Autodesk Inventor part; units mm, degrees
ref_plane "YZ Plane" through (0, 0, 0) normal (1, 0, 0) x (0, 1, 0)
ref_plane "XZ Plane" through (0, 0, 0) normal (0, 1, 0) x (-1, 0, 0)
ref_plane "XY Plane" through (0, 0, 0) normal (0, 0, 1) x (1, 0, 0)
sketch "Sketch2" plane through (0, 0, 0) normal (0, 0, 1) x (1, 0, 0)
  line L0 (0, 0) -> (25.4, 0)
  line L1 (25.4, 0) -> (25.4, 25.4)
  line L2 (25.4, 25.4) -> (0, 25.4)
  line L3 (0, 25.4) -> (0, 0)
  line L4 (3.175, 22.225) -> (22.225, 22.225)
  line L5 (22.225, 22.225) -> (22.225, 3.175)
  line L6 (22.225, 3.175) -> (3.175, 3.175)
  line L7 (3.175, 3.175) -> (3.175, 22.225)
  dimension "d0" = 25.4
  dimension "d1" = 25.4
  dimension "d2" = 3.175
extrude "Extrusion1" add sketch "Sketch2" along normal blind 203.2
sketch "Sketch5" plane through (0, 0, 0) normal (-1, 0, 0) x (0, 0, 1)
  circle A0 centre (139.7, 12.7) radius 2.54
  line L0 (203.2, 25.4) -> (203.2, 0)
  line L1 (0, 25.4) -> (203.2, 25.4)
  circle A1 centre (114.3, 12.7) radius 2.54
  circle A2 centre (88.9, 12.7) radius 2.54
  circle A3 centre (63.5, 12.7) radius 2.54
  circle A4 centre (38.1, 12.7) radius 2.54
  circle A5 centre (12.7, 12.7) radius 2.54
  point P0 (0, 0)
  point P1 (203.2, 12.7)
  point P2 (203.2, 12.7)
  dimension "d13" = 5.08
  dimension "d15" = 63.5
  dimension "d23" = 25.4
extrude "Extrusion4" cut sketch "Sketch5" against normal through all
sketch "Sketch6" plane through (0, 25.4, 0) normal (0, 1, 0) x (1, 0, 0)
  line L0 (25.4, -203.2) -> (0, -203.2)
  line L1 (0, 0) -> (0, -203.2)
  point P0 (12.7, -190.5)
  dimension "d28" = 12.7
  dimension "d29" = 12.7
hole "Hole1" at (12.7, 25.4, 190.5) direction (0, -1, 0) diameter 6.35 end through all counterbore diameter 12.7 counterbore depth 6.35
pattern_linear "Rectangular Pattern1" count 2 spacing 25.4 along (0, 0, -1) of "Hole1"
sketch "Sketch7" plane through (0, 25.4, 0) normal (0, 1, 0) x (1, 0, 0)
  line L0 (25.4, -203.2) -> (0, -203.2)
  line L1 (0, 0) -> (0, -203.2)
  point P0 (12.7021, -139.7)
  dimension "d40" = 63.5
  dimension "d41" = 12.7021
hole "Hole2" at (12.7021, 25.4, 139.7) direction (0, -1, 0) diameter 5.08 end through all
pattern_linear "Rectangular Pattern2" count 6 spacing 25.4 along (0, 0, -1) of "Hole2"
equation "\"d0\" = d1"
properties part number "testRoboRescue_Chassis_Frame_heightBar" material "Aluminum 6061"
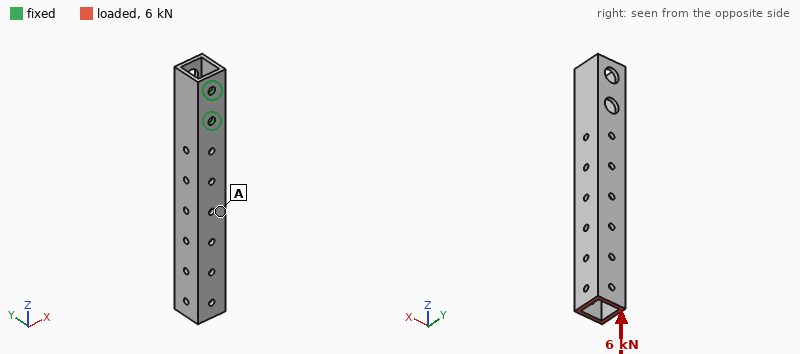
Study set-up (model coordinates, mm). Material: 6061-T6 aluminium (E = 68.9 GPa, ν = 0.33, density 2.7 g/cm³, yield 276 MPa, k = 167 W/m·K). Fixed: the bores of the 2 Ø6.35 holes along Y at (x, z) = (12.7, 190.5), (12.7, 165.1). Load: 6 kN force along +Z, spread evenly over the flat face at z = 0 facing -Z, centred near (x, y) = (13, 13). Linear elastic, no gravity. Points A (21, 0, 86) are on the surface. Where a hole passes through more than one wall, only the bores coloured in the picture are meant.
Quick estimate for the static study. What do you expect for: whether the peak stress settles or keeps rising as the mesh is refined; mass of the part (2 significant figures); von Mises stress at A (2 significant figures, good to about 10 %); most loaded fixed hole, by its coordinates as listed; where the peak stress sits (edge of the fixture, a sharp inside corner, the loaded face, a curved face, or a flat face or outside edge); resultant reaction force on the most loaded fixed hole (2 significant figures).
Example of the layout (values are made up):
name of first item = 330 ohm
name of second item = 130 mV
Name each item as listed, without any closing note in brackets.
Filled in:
whether the peak stress settles or keeps rising as the mesh is refined = keeps rising
mass of the part = 150 g
von Mises stress at A = 24 MPa
most loaded fixed hole, by its coordinates as listed = (12.7, 165.1)
where the peak stress sits = edge of the fixture
resultant reaction force on the most loaded fixed hole = 4.3 kN
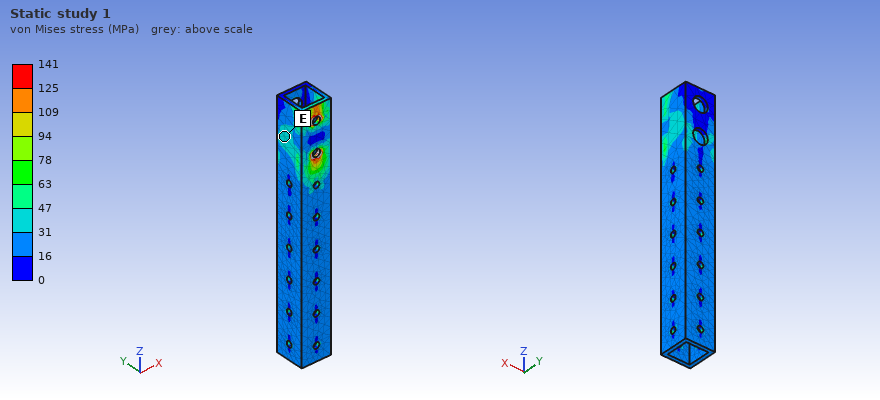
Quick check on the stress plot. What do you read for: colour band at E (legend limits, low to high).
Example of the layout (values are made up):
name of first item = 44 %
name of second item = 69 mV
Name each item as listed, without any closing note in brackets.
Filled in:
colour band at E = 31 to 47 MPa
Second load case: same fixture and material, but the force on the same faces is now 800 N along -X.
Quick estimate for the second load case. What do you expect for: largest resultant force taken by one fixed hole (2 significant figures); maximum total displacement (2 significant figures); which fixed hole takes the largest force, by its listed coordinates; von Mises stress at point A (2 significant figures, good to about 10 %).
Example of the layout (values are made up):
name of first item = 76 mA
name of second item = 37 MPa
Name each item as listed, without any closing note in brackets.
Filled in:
largest resultant force taken by one fixed hole = 4.5 kN
maximum total displacement = 1.5 mm
which fixed hole takes the largest force, by its listed coordinates = (12.7, 165.1)
von Mises stress at point A = 22 MPa
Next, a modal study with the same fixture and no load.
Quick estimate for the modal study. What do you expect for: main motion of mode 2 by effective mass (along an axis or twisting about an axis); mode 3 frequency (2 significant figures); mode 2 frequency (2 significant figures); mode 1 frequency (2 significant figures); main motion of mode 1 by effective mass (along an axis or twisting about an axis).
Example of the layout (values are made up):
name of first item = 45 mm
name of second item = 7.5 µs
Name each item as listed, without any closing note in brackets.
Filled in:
main motion of mode 2 by effective mass = along X
mode 3 frequency = 1700 Hz
mode 2 frequency = 630 Hz
mode 1 frequency = 500 Hz
main motion of mode 1 by effective mass = along Y
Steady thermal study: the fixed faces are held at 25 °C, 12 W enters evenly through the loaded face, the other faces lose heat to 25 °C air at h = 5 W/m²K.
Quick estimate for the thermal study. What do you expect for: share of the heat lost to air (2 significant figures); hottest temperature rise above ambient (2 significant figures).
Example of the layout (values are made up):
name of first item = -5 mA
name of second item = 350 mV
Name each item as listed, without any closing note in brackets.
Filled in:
share of the heat lost to air = 26 %
hottest temperature rise above ambient = 41 K
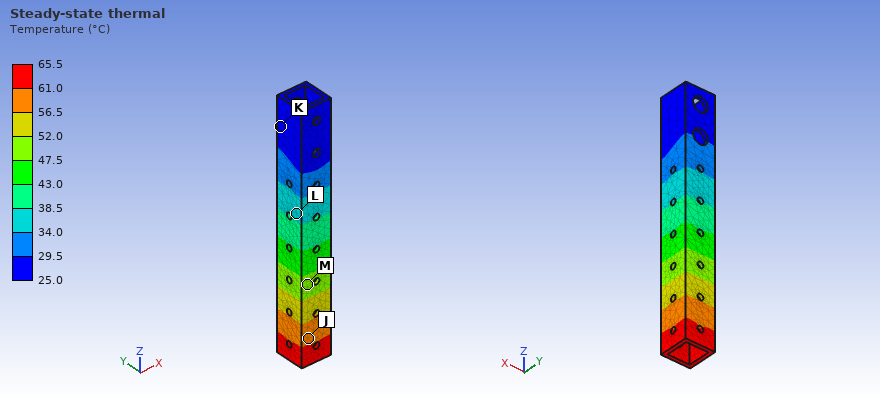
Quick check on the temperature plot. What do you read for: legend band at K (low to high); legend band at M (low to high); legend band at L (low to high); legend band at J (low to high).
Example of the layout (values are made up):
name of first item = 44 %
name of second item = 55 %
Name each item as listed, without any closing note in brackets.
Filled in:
legend band at K = 25.0 to 29.5 °C
legend band at M = 47.5 to 52.0 °C
legend band at L = 34.0 to 38.5 °C
legend band at J = 56.5 to 61.0 °C
